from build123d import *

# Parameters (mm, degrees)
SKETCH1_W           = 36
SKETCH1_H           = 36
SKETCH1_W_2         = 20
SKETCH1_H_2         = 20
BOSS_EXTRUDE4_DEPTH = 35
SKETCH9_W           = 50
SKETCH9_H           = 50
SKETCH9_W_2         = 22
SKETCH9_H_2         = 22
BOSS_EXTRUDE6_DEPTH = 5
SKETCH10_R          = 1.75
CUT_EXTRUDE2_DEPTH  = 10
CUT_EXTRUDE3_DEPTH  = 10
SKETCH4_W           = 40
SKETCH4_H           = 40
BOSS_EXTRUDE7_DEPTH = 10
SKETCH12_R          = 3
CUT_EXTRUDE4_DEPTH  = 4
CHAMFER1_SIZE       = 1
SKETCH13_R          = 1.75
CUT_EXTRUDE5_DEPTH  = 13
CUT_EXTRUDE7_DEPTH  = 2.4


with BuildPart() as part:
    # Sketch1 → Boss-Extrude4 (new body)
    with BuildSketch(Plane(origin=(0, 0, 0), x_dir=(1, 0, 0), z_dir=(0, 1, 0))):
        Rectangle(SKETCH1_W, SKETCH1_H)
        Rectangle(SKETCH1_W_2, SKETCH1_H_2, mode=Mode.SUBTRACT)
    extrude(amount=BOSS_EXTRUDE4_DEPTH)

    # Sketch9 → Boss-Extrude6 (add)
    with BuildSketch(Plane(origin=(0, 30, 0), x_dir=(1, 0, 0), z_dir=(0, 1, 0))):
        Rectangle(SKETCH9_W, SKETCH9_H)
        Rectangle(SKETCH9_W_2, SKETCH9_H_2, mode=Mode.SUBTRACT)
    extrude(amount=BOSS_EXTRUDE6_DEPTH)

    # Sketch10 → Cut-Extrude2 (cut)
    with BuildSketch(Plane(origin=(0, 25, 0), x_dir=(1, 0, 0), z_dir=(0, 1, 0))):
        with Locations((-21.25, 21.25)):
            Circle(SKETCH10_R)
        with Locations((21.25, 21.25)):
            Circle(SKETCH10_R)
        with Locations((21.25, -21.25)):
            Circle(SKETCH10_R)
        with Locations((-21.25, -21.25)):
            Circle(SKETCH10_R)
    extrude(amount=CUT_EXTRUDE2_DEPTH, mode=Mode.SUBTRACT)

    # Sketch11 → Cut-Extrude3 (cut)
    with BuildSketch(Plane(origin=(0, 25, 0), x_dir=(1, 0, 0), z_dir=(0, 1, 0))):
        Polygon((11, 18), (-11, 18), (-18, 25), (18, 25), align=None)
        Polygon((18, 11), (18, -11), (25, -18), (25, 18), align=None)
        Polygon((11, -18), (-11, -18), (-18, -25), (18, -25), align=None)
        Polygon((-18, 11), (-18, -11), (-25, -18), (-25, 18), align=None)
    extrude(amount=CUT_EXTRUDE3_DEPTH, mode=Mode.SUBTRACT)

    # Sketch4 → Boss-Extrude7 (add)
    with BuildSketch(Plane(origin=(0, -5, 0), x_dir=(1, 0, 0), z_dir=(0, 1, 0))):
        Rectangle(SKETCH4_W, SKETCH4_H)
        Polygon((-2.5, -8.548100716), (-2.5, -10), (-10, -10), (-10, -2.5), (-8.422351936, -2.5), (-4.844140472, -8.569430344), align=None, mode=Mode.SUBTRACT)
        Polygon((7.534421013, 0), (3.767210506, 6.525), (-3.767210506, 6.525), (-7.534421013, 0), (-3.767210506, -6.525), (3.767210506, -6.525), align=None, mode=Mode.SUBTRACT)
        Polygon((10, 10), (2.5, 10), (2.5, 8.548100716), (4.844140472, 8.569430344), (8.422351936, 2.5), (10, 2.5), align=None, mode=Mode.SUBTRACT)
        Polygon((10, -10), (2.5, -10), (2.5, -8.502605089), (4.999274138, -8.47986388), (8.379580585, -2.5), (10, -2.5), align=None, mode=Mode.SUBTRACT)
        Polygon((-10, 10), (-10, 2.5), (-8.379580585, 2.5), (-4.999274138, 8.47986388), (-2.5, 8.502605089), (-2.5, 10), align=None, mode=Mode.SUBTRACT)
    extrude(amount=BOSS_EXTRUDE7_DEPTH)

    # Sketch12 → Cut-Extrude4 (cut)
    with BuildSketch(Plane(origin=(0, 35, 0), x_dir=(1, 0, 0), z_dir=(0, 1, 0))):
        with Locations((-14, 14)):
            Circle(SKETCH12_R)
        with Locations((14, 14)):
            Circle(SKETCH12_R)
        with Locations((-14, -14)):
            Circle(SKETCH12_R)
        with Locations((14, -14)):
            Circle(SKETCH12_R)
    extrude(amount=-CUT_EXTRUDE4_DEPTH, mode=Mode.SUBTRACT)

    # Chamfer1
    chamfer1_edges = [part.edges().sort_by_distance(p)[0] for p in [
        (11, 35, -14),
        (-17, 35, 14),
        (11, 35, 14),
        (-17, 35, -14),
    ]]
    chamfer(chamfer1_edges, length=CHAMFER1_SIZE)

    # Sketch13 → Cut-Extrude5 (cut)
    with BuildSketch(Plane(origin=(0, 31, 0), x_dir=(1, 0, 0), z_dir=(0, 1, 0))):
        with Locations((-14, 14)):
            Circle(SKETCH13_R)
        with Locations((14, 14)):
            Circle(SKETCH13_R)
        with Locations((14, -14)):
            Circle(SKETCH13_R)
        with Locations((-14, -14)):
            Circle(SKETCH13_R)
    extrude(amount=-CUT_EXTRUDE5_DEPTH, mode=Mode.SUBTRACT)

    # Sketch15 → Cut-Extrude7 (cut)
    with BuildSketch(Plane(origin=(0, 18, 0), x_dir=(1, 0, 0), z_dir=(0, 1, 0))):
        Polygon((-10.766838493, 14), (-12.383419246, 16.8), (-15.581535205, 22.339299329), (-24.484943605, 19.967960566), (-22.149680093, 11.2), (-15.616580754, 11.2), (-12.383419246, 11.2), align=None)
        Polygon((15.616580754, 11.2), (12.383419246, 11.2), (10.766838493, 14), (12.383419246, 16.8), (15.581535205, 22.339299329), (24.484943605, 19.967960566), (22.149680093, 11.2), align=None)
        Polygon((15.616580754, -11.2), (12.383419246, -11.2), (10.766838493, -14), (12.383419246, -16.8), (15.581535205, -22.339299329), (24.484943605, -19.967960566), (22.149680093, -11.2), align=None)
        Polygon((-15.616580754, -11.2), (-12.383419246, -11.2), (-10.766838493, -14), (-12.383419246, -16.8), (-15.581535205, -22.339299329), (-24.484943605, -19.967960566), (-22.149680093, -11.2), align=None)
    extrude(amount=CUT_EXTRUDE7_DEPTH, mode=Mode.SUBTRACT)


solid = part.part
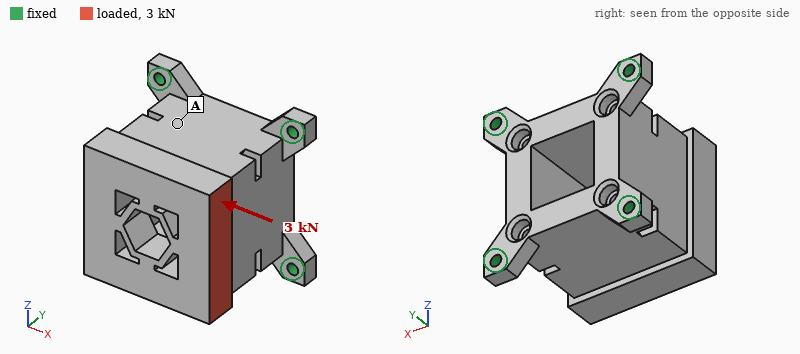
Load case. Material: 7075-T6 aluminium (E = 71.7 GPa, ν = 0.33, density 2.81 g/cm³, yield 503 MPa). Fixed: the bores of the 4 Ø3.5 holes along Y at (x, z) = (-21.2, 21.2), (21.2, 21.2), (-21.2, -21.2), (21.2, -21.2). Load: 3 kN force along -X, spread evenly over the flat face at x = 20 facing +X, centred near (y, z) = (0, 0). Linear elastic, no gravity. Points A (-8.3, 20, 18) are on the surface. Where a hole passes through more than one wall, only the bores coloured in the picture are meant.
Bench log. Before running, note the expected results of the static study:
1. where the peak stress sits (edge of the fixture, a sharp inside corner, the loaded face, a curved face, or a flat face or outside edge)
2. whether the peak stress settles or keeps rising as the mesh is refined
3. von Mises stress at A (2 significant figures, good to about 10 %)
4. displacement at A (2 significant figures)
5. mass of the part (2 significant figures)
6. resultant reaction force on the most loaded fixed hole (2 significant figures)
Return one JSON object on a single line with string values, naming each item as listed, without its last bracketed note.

{"where the peak stress sits": "edge of the fixture", "whether the peak stress settles or keeps rising as the mesh is refined": "keeps rising", "von Mises stress at A": "18 MPa", "displacement at A": "19 µm", "mass of the part": "110 g", "resultant reaction force on the most loaded fixed hole": "1.6 kN"}
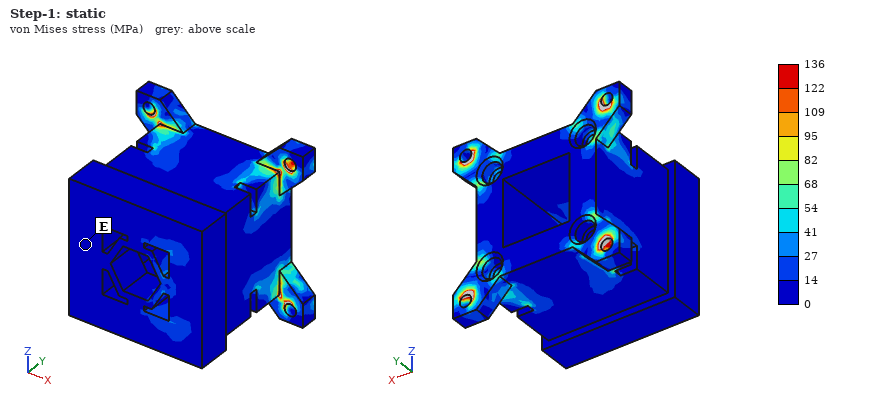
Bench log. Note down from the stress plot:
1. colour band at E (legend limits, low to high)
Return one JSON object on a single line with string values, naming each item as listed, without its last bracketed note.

{"colour band at E": "0 to 14 MPa"}
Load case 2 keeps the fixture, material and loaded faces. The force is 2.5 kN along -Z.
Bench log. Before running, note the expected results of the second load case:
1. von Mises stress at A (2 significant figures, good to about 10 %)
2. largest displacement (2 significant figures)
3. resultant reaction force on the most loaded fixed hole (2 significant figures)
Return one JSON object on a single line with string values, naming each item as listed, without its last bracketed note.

{"von Mises stress at A": "21 MPa", "largest displacement": "65 µm", "resultant reaction force on the most loaded fixed hole": "1.5 kN"}
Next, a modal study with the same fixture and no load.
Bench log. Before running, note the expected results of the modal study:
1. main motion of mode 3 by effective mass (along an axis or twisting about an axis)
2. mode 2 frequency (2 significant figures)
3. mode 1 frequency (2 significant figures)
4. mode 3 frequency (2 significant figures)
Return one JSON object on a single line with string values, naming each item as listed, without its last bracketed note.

{"main motion of mode 3 by effective mass": "along Y", "mode 2 frequency": "5000 Hz", "mode 1 frequency": "5000 Hz", "mode 3 frequency": "7300 Hz"}
